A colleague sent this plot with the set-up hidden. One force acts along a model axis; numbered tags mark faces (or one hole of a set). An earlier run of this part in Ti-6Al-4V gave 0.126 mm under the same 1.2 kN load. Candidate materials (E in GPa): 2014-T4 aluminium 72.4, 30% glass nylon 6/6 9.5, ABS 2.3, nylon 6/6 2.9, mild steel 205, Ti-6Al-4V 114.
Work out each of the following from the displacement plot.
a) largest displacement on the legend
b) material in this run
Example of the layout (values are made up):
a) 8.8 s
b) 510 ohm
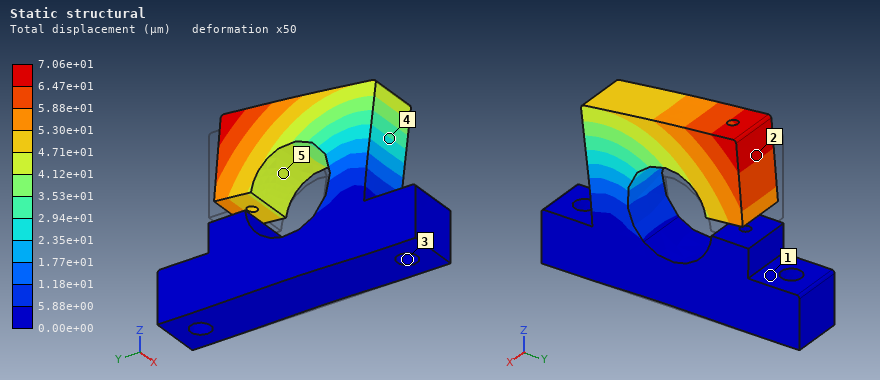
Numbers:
a) 7.06e+01 µm
b) mild steel
